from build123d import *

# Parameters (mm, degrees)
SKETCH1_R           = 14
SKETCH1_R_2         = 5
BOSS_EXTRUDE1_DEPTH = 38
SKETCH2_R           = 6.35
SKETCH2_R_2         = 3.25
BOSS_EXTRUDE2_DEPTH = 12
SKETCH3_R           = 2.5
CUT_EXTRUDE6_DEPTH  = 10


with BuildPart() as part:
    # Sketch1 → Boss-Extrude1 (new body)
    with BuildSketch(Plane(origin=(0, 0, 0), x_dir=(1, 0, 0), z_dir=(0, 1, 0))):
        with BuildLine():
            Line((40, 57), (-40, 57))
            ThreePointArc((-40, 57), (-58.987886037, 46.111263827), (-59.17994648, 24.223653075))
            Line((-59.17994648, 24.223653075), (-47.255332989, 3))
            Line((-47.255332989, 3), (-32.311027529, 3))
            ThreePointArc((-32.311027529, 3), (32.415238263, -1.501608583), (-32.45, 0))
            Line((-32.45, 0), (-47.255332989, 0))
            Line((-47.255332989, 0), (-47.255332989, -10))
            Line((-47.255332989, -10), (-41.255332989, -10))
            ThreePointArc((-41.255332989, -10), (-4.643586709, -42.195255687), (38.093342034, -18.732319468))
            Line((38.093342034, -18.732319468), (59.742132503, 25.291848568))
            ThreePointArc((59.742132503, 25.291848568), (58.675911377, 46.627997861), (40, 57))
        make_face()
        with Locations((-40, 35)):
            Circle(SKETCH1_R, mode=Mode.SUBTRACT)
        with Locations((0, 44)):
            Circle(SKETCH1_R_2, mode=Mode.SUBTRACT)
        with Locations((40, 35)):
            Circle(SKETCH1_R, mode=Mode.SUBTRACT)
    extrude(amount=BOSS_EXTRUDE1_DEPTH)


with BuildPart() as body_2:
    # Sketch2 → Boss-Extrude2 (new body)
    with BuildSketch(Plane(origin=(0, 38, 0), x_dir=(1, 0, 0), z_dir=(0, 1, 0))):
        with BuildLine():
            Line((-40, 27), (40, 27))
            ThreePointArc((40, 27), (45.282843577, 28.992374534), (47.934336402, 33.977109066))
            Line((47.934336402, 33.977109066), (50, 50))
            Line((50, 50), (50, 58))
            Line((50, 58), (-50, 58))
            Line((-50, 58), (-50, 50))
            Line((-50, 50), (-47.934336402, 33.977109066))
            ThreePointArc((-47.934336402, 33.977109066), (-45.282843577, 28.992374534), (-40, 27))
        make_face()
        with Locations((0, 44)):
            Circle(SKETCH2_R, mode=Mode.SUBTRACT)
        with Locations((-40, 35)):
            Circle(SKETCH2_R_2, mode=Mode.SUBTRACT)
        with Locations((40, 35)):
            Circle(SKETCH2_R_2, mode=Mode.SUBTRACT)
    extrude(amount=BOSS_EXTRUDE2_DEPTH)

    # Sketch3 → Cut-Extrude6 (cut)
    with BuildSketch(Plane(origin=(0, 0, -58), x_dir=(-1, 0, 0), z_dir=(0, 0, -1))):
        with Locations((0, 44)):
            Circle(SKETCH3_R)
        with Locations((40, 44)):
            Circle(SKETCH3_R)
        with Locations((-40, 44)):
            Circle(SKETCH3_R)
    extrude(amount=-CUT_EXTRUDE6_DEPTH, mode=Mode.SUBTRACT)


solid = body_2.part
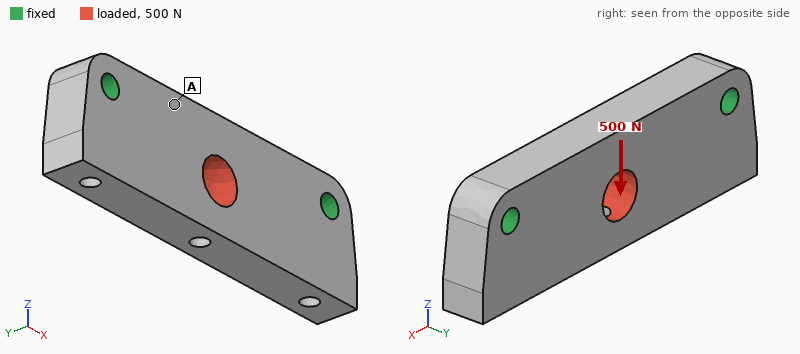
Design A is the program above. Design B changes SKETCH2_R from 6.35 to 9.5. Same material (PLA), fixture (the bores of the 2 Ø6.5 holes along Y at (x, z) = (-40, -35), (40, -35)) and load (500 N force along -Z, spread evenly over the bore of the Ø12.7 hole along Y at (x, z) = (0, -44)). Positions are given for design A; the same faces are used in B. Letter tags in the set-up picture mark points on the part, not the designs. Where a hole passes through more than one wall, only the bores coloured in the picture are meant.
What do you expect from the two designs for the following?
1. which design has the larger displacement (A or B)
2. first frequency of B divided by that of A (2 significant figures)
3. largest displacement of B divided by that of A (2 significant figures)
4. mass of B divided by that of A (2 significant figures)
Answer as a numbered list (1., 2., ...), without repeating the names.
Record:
1. B
2. 1.0
3. 1.1
4. 0.95
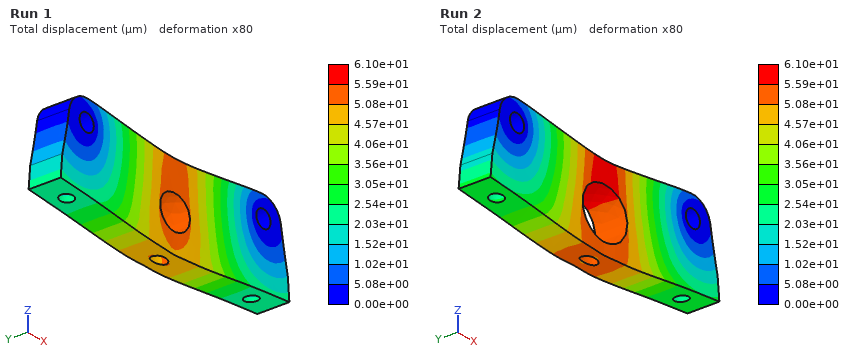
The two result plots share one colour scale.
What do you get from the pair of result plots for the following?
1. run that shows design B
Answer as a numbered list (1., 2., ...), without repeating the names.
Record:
1. Run 2
